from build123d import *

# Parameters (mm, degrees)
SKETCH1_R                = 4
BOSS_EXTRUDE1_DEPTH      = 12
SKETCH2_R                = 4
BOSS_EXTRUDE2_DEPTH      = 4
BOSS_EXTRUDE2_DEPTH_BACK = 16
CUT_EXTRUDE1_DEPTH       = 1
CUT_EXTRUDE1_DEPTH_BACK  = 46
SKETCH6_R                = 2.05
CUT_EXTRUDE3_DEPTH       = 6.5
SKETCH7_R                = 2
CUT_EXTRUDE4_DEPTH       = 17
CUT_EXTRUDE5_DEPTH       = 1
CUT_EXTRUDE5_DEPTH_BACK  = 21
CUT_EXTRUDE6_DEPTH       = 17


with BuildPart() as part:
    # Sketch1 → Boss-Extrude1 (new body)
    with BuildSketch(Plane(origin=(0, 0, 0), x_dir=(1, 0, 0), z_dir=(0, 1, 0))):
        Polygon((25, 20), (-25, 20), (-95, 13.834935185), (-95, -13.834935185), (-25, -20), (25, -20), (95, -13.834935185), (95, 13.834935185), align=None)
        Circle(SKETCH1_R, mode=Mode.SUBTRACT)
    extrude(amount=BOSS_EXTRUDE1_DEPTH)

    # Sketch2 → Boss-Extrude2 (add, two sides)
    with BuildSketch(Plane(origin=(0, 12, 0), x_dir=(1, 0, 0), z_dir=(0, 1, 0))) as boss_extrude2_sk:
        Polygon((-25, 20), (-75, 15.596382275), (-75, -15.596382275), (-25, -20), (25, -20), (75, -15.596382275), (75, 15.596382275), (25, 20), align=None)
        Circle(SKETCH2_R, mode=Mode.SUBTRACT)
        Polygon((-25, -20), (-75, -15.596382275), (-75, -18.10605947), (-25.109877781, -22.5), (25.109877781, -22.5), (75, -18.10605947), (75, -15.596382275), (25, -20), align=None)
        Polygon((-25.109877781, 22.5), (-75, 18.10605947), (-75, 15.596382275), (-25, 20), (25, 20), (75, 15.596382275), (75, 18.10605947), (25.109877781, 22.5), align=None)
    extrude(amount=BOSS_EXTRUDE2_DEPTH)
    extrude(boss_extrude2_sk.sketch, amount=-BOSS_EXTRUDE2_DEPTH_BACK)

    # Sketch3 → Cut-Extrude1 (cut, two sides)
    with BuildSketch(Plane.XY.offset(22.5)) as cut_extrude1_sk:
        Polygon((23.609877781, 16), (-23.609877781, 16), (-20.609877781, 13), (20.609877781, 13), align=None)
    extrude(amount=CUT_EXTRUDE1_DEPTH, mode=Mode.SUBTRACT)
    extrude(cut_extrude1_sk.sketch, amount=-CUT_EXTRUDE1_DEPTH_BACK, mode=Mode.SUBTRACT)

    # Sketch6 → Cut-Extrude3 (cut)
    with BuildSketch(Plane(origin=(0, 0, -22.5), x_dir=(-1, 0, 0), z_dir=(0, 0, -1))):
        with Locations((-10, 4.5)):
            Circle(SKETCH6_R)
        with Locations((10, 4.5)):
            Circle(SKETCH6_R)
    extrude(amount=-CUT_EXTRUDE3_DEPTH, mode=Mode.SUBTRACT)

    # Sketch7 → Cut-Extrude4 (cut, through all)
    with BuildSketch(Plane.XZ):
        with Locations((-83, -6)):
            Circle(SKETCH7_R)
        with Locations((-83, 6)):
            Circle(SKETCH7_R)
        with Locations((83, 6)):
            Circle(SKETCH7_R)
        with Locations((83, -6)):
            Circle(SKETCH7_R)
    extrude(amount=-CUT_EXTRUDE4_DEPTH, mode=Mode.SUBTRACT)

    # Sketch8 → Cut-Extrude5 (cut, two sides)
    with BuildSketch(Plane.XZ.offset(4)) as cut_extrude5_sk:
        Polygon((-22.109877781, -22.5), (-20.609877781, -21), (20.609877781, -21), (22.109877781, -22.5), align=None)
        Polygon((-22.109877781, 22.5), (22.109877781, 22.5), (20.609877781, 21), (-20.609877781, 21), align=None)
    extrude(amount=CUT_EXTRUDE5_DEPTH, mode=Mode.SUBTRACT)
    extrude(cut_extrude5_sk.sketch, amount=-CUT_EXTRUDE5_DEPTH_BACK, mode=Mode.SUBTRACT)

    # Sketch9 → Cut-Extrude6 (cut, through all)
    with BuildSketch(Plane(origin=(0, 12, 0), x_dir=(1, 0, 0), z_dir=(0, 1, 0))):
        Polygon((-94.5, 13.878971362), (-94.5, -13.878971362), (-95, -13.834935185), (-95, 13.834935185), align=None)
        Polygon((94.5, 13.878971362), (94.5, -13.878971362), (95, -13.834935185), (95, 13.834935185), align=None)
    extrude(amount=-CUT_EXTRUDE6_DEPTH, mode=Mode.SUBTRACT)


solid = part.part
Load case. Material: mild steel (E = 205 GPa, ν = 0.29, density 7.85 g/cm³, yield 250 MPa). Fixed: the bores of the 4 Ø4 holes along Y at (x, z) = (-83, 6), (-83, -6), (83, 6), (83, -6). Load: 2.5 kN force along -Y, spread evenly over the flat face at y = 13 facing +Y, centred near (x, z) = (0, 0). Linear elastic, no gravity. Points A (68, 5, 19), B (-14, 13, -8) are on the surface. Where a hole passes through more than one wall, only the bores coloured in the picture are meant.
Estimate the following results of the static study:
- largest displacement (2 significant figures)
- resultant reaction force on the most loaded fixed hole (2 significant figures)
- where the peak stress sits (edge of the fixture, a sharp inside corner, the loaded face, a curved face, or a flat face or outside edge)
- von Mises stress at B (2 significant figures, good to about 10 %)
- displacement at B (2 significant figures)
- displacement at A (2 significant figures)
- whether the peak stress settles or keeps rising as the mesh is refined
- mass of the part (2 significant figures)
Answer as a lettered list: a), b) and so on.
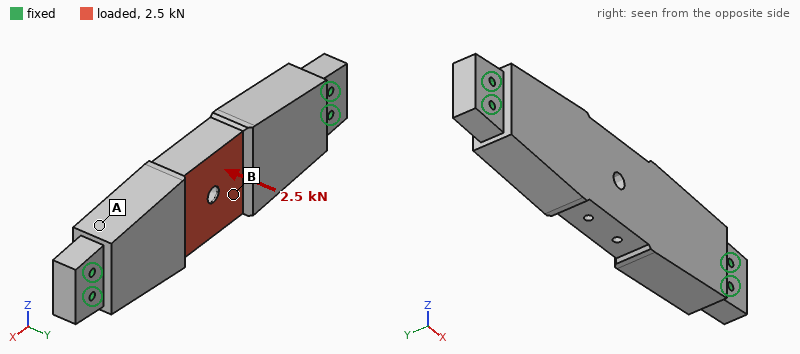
a) 29 µm
b) 730 N
c) edge of the fixture
d) 21 MPa
e) 26 µm
f) 4.6 µm
g) keeps rising
h) 1.0 kg
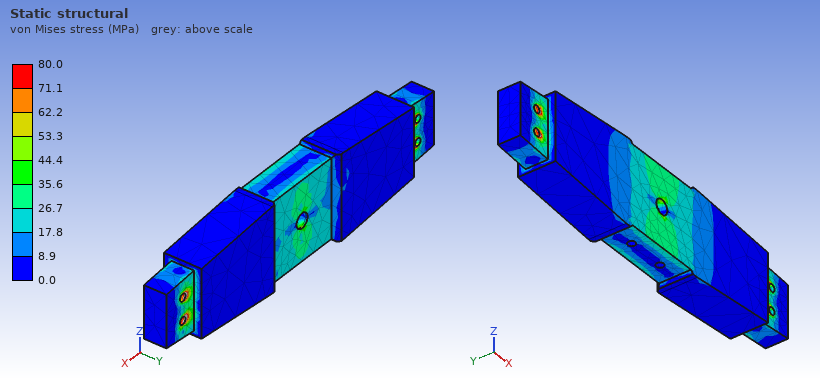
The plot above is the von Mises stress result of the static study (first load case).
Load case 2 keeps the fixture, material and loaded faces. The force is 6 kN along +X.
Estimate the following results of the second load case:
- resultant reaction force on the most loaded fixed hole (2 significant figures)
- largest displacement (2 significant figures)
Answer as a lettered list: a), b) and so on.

a) 1.5 kN
b) 2.5 µm
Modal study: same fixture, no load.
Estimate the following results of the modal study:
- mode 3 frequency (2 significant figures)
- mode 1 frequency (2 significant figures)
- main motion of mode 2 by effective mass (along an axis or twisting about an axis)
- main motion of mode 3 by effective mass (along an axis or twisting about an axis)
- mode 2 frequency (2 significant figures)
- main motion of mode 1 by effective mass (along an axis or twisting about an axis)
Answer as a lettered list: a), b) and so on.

a) 5300 Hz
b) 2200 Hz
c) along Z
d) twisting about X
e) 4200 Hz
f) along Y
